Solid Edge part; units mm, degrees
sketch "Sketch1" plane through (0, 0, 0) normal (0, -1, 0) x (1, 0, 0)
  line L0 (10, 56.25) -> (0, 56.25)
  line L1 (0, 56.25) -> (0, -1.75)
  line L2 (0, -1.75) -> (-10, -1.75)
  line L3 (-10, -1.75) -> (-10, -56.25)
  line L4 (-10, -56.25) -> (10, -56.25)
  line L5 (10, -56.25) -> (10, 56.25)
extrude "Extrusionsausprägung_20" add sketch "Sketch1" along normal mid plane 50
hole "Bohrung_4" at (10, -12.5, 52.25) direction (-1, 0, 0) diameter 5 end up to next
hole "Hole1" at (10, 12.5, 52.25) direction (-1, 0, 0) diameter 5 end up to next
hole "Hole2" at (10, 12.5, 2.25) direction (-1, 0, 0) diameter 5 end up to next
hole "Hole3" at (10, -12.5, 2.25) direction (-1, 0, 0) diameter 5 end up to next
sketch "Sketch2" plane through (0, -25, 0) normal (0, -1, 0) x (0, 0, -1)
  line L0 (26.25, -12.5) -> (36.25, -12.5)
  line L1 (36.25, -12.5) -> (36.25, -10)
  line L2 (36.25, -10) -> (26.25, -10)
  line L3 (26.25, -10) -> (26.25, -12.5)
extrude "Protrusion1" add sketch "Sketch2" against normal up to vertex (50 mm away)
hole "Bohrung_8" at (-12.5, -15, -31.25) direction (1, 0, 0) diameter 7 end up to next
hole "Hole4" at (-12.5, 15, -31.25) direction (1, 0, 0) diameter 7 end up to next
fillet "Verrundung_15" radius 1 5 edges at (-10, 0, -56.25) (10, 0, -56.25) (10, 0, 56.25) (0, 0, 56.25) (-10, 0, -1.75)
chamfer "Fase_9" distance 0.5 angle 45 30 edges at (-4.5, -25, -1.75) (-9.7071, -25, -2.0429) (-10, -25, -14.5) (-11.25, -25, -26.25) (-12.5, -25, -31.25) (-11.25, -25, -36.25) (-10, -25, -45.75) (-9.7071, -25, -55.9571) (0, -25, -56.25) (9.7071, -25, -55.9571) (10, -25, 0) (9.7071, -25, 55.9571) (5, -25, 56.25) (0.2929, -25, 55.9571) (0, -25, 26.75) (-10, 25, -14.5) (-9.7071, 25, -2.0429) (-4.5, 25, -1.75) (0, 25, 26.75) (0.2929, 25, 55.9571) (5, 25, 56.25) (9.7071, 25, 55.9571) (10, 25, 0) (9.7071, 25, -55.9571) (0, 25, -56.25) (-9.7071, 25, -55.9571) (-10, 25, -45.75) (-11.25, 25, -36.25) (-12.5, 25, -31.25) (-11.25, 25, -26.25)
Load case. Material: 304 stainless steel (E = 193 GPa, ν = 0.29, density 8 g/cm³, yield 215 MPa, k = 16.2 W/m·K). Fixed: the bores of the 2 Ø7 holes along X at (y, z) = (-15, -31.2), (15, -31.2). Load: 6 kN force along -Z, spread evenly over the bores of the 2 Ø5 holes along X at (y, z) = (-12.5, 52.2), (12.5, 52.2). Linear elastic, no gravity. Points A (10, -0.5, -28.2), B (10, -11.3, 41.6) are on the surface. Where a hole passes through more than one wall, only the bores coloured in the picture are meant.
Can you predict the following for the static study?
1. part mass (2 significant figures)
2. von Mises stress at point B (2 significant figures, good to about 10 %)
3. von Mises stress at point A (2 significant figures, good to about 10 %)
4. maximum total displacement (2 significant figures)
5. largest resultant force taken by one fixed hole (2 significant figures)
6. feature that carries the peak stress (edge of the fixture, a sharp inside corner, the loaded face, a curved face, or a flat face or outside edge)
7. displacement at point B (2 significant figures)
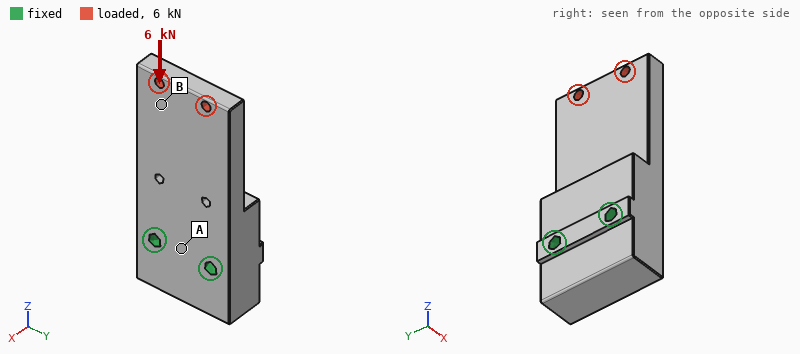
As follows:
660 g
17 MPa
7.0 MPa
13 µm
3.0 kN
a curved face
9.5 µm
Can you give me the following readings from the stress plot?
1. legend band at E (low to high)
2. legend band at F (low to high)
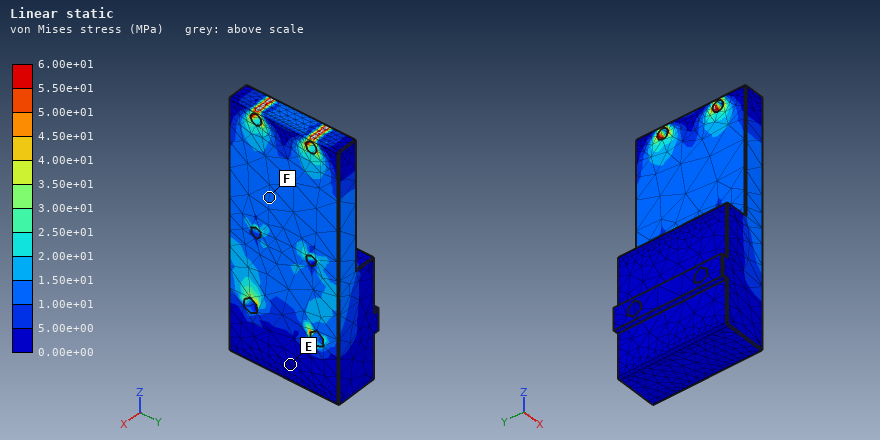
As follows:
0.00e+00 to 5.00e+00 MPa
1.00e+01 to 1.50e+01 MPa
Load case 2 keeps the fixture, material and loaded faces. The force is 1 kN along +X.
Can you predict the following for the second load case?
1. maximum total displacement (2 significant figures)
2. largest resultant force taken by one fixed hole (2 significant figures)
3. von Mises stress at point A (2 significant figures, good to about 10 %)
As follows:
0.12 mm
500 N
12 MPa
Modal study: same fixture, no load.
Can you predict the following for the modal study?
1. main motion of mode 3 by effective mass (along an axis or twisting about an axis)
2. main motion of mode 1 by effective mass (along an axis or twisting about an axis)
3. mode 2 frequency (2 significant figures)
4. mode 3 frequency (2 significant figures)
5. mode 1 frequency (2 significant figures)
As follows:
along Y
along X
4800 Hz
5100 Hz
1700 Hz
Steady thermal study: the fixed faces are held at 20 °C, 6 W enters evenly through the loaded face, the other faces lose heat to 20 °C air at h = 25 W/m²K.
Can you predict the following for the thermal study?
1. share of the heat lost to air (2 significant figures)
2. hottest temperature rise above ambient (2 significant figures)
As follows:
60 %
35 K
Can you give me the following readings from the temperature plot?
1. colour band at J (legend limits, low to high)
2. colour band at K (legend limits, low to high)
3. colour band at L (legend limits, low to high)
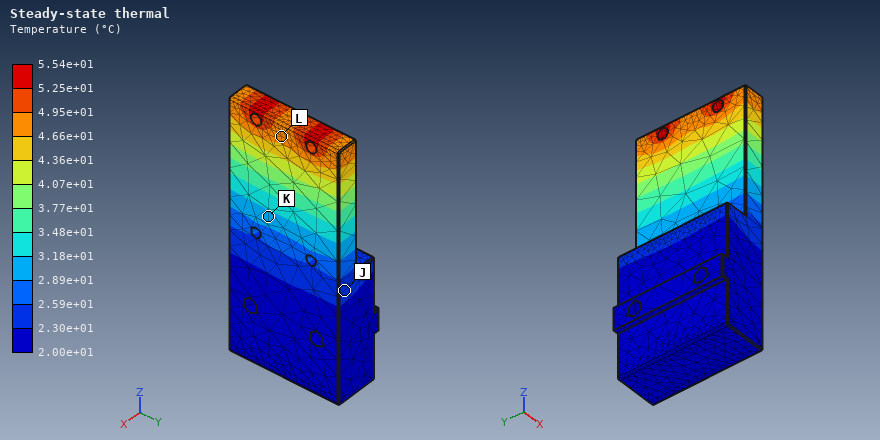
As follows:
2.30e+01 to 2.59e+01 °C
2.89e+01 to 3.18e+01 °C
4.66e+01 to 4.95e+01 °C
